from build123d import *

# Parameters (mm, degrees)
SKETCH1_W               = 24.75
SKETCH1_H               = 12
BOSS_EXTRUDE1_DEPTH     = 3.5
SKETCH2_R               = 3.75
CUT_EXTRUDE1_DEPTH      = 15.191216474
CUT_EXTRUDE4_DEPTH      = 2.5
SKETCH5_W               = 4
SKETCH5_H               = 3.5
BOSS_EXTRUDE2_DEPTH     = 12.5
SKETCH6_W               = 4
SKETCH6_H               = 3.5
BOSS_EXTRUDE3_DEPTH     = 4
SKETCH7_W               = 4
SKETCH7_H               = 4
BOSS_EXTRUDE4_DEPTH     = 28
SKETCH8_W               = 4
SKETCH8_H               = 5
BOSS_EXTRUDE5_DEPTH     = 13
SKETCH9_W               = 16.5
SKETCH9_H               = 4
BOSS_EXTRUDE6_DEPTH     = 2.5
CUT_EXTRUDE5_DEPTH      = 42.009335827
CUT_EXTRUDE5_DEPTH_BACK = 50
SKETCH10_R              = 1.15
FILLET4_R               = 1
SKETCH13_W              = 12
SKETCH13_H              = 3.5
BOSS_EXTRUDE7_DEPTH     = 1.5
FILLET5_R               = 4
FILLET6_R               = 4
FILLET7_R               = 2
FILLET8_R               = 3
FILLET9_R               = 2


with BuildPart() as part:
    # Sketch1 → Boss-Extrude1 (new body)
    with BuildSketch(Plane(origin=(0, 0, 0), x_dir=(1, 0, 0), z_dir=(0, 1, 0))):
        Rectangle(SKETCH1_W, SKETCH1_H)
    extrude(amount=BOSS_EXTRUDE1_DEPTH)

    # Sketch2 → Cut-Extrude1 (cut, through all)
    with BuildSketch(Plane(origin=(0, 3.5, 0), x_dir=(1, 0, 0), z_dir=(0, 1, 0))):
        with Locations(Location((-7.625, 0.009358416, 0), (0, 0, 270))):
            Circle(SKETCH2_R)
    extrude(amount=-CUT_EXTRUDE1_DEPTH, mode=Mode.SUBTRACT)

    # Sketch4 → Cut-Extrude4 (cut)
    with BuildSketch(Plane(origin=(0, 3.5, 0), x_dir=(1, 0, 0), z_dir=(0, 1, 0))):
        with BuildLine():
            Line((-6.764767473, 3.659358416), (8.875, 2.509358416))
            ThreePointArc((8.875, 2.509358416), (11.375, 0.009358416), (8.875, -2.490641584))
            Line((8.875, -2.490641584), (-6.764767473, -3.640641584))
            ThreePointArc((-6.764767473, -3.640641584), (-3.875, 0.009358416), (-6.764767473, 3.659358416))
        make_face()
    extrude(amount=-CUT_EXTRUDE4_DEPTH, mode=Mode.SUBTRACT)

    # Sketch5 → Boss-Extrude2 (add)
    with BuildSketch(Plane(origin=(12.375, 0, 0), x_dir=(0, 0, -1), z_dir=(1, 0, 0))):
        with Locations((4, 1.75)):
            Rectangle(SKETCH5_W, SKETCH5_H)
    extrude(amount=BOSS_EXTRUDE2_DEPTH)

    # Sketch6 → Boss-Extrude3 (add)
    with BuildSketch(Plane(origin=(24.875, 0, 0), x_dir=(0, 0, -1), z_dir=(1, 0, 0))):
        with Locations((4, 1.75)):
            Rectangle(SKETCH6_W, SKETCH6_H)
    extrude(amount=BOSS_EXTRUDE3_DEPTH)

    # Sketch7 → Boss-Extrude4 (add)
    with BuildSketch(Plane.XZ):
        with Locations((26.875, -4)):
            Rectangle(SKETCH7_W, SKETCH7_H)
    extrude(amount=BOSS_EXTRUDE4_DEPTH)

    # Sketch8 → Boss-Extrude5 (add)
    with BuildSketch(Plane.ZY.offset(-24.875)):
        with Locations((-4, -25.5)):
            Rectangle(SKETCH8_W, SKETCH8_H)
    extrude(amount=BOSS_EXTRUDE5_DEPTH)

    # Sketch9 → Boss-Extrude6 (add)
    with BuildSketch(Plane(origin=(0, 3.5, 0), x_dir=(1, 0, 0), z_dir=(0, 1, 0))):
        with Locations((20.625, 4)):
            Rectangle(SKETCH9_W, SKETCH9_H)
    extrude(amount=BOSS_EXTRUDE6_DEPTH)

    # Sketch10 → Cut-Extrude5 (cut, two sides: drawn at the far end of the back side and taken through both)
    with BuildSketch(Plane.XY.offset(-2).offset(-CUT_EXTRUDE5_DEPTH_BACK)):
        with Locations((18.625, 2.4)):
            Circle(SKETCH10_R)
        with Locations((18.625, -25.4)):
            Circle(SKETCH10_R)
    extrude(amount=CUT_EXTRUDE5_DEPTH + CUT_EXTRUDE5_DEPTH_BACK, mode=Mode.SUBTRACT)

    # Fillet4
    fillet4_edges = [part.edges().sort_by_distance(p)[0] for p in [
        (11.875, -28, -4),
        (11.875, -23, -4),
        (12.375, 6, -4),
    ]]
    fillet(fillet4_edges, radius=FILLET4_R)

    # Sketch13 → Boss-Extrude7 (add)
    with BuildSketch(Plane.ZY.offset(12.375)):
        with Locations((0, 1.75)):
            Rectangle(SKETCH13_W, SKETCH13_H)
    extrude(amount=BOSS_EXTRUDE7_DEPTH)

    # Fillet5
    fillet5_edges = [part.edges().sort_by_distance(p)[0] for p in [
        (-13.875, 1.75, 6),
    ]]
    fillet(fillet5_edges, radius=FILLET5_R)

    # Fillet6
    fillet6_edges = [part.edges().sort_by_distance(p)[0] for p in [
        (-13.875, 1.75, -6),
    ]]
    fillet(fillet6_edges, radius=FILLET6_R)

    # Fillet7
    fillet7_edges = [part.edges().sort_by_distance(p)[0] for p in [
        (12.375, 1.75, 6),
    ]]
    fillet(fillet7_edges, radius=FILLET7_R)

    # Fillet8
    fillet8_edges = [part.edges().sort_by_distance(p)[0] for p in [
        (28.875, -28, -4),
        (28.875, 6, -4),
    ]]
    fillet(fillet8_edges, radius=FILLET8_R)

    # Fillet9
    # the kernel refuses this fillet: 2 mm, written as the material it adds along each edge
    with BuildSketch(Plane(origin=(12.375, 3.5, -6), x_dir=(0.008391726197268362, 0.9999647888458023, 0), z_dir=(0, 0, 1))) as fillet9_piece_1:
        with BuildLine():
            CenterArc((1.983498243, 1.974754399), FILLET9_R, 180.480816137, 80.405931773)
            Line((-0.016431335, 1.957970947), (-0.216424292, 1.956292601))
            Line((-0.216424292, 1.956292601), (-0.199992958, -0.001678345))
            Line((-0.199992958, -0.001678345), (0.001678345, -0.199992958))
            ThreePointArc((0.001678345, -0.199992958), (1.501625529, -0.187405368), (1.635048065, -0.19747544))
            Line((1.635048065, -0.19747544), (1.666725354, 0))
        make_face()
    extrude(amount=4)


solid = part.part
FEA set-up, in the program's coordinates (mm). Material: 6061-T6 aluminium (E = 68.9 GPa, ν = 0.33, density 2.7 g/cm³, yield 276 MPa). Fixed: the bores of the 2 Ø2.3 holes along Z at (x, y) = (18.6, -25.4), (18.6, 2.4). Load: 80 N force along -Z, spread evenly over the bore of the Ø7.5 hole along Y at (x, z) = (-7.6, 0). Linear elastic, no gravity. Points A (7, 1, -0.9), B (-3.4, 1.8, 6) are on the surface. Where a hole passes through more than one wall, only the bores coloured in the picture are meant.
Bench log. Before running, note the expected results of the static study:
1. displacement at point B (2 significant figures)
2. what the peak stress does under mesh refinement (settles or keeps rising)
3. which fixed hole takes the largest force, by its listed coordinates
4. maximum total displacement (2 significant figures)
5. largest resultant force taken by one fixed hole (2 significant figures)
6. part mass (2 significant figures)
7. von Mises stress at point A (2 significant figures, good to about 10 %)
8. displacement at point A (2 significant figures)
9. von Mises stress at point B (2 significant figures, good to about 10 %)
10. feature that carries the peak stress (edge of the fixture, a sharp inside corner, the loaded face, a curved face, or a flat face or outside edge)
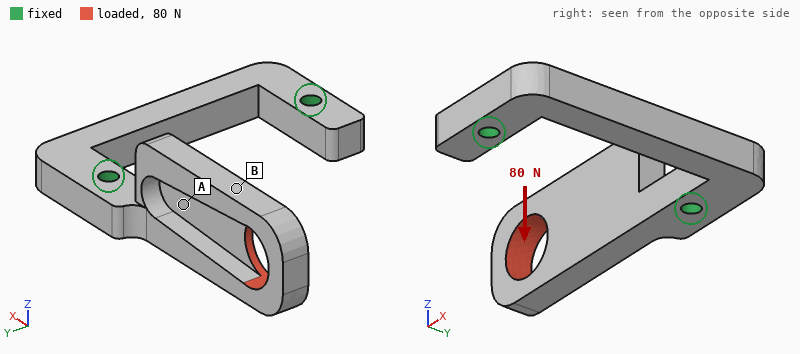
0.20 mm
keeps rising
(18.6, 2.4)
0.30 mm
80 N
4.7 g
45 MPa
0.071 mm
17 MPa
edge of the fixture
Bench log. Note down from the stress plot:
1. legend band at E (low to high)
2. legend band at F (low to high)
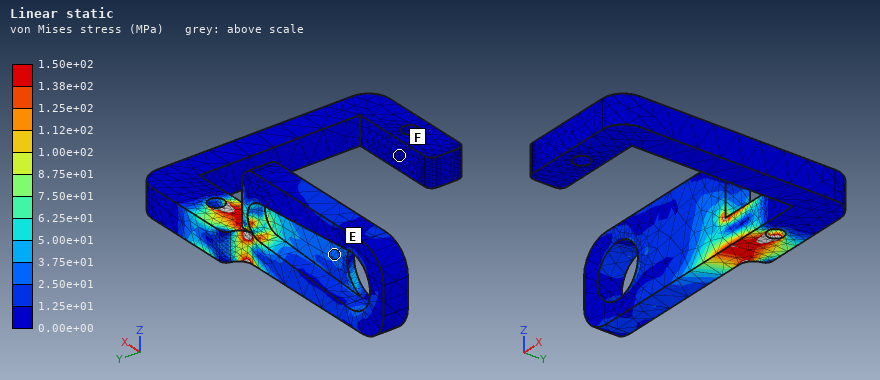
2.50e+01 to 3.75e+01 MPa
0.00e+00 to 1.25e+01 MPa
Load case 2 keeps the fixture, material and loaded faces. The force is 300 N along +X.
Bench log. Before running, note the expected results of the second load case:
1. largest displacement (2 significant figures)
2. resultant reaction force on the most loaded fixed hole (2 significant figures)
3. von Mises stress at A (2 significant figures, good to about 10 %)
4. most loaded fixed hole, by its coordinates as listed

0.18 mm
300 N
43 MPa
(18.6, 2.4)
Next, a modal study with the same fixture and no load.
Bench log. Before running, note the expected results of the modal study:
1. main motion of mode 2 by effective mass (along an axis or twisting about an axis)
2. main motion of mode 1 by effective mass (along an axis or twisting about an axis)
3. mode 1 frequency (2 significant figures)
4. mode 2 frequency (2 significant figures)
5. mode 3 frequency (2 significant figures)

along Z
along Y
2600 Hz
2900 Hz
7500 Hz
